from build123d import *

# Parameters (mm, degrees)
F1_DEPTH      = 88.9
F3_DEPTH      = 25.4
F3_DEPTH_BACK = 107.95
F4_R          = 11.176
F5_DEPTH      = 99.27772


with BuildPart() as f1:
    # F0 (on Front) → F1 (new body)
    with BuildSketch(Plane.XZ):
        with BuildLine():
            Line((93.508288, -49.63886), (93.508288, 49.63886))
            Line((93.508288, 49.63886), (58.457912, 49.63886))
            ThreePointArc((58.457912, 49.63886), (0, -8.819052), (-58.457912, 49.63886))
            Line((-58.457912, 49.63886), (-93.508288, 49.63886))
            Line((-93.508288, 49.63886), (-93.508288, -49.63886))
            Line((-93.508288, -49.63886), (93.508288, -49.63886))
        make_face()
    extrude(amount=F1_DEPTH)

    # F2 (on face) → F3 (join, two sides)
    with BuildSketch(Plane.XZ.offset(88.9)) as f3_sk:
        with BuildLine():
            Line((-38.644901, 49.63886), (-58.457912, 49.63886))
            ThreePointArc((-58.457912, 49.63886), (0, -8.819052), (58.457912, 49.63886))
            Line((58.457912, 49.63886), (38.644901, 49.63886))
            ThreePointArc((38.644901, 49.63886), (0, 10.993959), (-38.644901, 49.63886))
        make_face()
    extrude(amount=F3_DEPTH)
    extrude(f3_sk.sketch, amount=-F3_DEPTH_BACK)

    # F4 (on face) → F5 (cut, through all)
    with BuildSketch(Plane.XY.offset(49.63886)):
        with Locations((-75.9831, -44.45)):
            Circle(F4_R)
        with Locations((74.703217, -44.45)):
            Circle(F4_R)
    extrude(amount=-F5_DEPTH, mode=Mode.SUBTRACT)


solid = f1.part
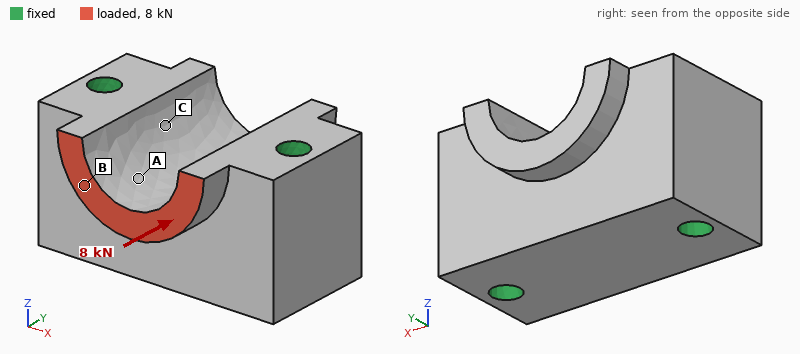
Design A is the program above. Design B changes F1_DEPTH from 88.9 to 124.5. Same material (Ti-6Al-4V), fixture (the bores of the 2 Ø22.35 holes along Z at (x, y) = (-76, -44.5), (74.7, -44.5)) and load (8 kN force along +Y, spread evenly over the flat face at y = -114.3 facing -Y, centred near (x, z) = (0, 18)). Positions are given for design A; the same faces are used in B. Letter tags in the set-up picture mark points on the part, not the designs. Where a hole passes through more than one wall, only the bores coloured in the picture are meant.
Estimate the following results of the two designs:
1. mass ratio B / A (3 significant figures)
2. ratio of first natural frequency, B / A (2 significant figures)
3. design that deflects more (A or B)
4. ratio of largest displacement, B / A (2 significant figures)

1.31
0.82
A
0.74
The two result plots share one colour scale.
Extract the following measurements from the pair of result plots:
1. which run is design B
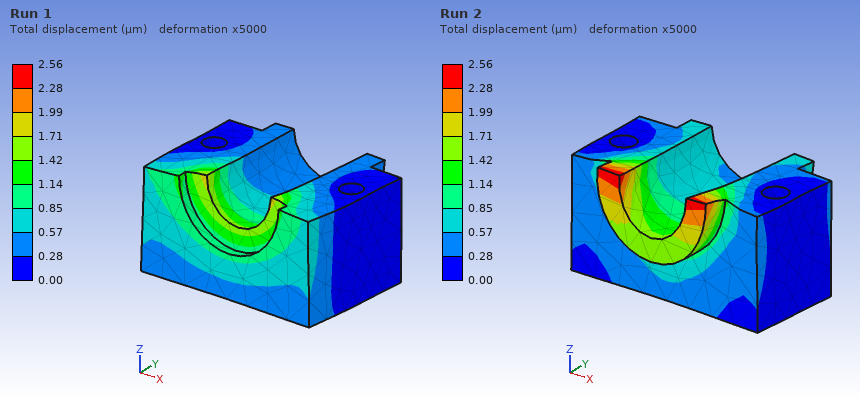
Run 1
